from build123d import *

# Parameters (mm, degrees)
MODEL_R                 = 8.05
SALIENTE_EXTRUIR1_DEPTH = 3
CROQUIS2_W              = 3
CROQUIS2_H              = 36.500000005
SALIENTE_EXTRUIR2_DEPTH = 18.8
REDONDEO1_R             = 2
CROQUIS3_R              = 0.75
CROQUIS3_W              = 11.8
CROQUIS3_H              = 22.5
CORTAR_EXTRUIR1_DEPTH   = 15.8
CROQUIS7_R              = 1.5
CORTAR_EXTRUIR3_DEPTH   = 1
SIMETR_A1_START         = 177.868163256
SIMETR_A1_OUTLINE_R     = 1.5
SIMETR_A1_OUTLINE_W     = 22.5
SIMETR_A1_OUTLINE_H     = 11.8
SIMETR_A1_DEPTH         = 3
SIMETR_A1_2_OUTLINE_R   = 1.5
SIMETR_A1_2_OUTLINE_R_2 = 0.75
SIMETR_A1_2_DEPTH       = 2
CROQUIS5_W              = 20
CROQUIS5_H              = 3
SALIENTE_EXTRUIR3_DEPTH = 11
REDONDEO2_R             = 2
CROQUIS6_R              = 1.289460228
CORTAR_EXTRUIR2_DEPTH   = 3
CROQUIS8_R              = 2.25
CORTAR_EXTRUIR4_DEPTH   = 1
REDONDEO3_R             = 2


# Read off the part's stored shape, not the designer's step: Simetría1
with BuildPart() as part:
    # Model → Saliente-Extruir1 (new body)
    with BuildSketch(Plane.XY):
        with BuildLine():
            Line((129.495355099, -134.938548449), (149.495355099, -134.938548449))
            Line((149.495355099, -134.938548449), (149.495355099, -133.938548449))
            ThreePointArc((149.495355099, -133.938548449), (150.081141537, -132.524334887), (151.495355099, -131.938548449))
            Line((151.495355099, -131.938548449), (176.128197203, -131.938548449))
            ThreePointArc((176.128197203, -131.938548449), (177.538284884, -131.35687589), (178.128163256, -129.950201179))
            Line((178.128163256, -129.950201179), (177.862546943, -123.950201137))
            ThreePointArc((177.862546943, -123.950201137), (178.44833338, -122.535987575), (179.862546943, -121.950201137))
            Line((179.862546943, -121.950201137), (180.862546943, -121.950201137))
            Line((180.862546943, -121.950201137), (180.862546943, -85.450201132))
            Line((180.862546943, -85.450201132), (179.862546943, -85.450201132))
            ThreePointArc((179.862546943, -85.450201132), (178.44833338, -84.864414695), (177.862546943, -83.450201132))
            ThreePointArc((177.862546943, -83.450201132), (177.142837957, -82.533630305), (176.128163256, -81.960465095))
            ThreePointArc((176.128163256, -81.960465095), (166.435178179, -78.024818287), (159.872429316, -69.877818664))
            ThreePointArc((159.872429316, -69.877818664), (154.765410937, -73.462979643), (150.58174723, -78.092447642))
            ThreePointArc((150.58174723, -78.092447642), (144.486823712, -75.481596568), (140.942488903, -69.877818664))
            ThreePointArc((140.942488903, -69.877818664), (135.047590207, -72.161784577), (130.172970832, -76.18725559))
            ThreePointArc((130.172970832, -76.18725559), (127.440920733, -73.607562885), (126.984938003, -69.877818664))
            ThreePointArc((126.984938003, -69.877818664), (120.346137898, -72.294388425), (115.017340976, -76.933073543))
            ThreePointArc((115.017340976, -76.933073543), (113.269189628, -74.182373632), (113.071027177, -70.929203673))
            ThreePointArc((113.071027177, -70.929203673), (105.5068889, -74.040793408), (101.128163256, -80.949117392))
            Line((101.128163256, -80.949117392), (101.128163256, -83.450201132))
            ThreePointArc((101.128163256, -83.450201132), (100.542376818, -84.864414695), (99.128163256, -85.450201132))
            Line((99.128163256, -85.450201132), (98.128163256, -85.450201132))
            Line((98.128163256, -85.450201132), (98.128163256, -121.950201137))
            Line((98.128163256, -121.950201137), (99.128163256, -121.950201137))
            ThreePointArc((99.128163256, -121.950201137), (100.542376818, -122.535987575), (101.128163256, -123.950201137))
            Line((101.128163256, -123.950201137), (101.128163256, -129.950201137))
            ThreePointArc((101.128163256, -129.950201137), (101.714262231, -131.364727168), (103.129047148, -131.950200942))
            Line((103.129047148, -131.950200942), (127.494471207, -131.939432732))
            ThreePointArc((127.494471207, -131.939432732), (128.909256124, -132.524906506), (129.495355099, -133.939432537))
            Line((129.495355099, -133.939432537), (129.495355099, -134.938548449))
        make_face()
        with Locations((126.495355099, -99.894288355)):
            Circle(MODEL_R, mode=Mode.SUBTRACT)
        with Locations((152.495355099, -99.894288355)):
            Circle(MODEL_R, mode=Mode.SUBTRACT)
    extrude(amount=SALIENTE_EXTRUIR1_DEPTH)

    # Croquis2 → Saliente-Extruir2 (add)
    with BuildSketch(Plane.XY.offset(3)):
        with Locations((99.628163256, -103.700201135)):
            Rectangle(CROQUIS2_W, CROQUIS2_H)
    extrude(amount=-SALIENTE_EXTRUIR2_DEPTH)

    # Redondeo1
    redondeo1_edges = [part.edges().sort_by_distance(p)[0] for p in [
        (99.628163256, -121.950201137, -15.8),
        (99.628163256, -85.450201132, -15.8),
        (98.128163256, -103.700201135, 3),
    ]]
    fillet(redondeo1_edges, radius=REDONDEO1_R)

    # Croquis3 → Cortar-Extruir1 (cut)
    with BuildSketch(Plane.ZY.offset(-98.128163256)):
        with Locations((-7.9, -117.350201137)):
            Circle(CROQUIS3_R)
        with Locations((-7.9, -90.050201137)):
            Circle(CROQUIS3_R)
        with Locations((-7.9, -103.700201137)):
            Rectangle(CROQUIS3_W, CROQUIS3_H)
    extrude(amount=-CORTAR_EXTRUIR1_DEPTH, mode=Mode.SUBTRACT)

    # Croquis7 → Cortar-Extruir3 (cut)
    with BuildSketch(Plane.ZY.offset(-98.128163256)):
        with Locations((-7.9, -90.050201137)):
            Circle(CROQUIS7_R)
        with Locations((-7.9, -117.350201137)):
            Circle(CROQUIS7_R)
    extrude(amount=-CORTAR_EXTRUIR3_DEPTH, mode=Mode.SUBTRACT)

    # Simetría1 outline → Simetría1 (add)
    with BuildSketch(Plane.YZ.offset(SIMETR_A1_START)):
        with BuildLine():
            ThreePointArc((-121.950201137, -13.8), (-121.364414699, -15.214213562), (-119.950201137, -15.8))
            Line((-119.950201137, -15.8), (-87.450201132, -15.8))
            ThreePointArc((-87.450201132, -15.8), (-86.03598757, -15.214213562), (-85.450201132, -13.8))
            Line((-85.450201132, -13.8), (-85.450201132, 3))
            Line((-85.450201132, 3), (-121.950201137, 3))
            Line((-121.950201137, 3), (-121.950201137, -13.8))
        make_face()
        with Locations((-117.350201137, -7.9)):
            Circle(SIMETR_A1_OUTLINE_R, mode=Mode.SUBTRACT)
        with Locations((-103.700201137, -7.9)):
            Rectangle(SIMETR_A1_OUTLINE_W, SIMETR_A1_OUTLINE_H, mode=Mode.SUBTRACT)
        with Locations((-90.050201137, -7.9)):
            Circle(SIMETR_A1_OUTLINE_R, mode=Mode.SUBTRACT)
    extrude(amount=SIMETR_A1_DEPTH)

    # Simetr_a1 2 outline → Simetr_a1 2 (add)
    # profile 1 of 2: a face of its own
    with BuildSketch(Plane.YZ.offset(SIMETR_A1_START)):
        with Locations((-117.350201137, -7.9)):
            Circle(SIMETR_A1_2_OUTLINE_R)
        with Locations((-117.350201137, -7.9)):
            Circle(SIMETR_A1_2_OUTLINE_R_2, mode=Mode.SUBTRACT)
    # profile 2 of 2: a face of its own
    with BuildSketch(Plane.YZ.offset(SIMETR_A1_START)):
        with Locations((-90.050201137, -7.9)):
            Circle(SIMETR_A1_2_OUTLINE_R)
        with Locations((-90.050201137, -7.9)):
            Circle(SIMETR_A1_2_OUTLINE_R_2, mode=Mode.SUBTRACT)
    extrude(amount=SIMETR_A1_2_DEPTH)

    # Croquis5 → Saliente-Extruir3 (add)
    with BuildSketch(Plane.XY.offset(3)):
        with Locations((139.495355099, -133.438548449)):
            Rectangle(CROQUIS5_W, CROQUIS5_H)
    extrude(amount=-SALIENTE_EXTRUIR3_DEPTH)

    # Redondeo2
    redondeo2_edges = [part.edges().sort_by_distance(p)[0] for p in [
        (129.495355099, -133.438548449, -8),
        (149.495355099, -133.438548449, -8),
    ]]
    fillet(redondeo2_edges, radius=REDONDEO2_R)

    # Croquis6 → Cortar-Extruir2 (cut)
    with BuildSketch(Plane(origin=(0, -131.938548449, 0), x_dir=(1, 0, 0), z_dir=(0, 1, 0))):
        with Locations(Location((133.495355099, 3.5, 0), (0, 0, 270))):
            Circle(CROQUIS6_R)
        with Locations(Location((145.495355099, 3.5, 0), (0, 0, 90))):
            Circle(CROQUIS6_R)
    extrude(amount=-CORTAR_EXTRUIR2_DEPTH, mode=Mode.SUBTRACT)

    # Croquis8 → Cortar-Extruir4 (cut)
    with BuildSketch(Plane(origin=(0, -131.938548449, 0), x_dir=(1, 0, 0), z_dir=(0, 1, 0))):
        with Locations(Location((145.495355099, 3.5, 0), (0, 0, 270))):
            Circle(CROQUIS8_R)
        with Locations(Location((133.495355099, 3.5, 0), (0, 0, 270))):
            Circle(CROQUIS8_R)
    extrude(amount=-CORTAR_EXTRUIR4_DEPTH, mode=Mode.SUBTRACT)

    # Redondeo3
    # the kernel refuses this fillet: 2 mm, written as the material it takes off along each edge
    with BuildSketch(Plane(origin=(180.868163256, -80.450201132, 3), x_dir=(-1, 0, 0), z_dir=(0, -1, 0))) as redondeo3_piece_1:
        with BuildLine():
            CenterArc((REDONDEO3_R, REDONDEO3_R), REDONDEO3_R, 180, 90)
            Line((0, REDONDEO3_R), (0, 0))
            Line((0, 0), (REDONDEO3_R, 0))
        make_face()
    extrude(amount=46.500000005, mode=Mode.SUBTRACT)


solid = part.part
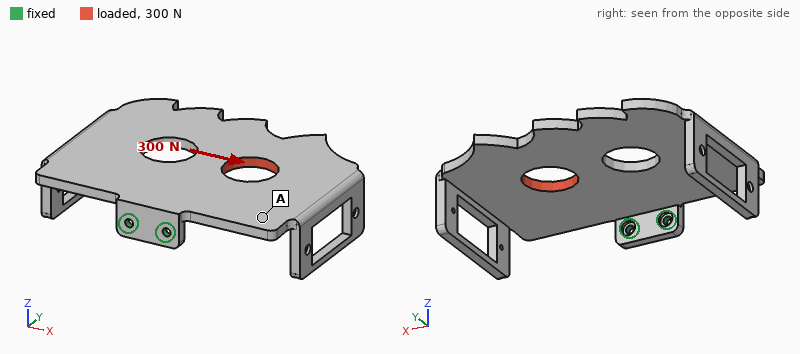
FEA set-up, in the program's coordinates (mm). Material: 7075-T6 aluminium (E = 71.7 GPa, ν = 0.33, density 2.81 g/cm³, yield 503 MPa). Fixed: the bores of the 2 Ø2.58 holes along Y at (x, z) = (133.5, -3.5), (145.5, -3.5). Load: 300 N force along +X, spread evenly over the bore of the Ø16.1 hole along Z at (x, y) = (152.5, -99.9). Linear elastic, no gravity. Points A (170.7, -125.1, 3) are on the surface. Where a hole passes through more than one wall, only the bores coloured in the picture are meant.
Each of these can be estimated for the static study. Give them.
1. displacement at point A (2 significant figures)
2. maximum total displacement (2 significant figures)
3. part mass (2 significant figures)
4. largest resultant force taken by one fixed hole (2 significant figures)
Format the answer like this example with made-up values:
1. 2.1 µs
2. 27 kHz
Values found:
1. 0.13 mm
2. 0.27 mm
3. 42 g
4. 780 N
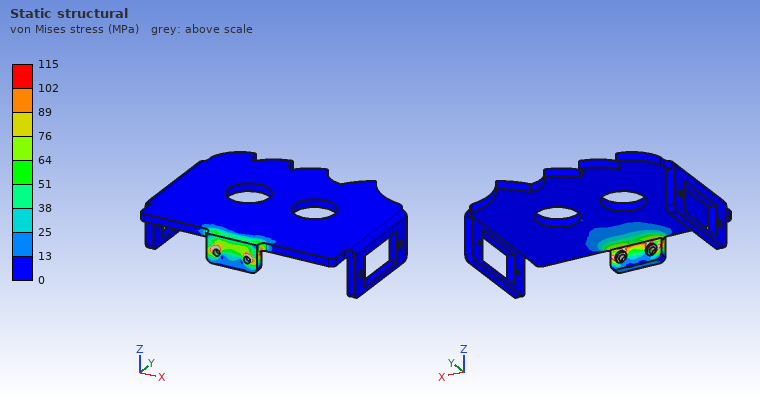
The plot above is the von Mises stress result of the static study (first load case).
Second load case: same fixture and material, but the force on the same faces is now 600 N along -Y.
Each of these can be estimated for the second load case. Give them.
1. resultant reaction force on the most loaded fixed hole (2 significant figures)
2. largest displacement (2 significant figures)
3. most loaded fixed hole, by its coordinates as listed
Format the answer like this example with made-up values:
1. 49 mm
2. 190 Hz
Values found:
1. 880 N
2. 0.35 mm
3. (145.5, -3.5)
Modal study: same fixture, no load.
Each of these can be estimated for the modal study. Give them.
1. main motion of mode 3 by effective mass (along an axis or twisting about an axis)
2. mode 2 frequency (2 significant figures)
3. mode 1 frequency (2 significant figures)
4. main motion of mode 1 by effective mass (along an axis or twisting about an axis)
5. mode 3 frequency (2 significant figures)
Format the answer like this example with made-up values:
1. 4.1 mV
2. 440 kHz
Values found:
1. along X
2. 580 Hz
3. 350 Hz
4. along Z
5. 1000 Hz
